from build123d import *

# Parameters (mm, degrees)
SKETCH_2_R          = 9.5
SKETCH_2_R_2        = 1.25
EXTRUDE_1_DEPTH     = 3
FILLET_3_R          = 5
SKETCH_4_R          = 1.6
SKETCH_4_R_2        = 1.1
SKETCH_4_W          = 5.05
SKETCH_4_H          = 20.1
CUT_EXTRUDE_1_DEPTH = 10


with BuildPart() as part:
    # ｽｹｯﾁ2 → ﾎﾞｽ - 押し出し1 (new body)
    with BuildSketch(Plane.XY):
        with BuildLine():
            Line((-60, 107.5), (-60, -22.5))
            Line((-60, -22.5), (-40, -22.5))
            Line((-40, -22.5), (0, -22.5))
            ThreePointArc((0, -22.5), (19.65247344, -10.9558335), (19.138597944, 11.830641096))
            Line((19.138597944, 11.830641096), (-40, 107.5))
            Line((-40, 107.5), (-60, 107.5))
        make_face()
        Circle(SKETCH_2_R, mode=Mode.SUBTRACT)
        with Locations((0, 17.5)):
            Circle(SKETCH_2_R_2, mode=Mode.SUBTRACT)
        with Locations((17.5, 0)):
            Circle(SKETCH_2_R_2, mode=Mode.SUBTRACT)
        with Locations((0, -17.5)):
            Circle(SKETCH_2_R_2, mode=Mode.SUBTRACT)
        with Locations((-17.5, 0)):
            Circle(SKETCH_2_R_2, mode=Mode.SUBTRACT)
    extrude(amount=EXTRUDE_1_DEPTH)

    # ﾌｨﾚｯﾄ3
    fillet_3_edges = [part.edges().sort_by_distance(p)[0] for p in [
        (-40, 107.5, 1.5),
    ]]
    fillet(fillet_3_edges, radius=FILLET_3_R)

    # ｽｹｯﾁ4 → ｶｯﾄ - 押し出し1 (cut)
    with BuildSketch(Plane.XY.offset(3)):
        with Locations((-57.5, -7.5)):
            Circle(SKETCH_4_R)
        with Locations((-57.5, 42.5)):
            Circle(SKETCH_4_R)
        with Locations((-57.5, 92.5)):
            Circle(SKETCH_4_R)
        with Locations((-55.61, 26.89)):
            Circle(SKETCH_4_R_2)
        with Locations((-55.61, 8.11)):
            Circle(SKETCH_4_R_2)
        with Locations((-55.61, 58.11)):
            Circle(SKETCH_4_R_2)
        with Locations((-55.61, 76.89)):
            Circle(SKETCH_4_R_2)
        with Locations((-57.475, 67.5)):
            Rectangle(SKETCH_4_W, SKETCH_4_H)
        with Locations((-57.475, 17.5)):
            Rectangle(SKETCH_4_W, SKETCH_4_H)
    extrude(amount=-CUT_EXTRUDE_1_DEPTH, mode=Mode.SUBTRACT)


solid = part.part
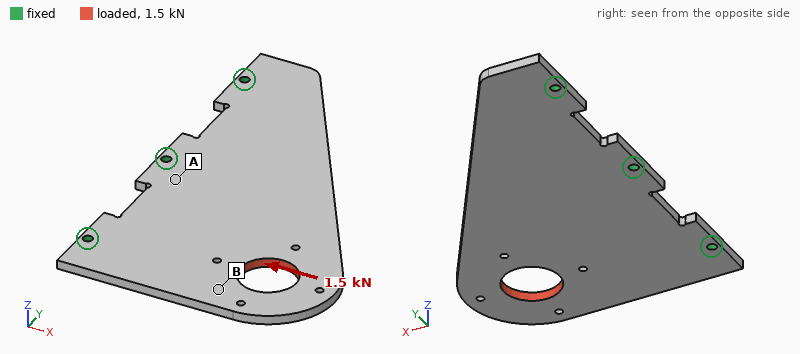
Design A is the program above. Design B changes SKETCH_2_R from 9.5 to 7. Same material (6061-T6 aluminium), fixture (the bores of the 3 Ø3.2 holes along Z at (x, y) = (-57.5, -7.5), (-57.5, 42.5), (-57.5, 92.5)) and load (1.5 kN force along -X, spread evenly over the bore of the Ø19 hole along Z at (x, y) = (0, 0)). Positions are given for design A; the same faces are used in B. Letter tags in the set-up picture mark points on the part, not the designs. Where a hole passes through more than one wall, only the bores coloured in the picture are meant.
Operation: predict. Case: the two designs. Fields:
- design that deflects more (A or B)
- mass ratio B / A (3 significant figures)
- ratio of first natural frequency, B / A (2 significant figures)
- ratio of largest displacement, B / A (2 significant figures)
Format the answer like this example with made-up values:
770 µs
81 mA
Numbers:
A
1.02
0.97
0.90
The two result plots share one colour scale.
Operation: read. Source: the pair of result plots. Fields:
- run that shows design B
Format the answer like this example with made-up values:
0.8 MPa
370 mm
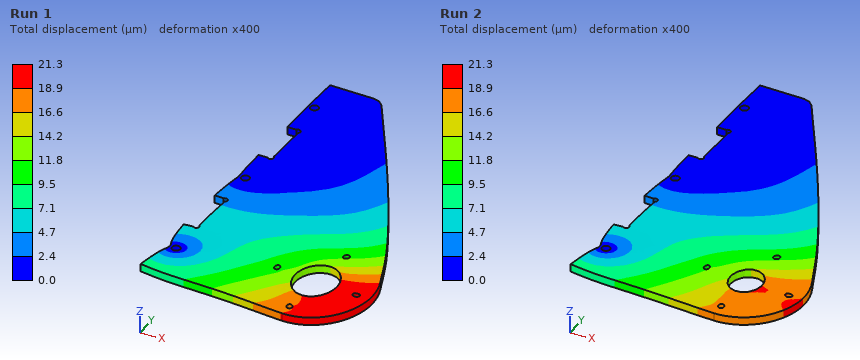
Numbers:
Run 2
